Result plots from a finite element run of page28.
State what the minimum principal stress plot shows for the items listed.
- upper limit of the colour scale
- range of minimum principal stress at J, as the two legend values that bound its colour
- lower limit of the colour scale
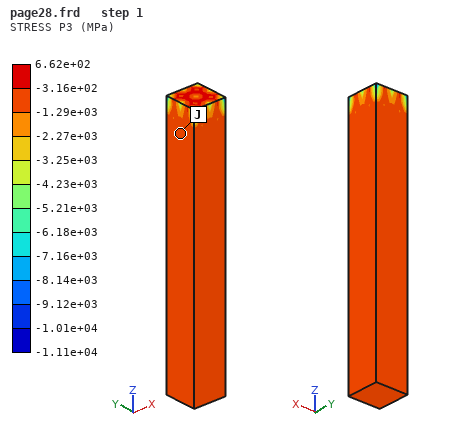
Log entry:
6.62e+02 MPa
-1.29e+03 to -3.16e+02 MPa
-1.11e+04 MPa
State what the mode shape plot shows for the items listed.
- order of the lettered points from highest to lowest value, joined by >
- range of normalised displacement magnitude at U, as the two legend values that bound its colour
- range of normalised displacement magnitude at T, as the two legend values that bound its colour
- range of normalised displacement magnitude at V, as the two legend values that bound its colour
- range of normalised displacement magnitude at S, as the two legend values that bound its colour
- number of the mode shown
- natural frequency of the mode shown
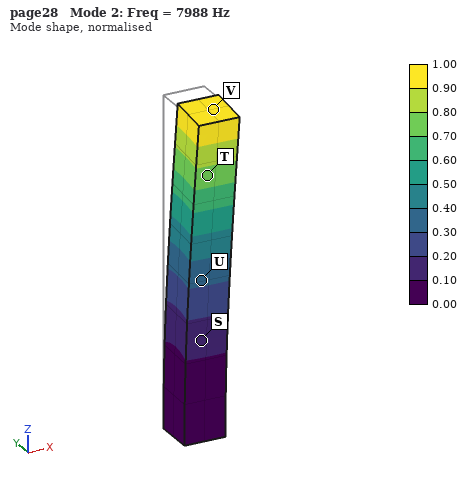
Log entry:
V > T > U > S
0.30 to 0.40
0.70 to 0.80
0.90 to 1.00
0.10 to 0.20
2
7988 Hz
